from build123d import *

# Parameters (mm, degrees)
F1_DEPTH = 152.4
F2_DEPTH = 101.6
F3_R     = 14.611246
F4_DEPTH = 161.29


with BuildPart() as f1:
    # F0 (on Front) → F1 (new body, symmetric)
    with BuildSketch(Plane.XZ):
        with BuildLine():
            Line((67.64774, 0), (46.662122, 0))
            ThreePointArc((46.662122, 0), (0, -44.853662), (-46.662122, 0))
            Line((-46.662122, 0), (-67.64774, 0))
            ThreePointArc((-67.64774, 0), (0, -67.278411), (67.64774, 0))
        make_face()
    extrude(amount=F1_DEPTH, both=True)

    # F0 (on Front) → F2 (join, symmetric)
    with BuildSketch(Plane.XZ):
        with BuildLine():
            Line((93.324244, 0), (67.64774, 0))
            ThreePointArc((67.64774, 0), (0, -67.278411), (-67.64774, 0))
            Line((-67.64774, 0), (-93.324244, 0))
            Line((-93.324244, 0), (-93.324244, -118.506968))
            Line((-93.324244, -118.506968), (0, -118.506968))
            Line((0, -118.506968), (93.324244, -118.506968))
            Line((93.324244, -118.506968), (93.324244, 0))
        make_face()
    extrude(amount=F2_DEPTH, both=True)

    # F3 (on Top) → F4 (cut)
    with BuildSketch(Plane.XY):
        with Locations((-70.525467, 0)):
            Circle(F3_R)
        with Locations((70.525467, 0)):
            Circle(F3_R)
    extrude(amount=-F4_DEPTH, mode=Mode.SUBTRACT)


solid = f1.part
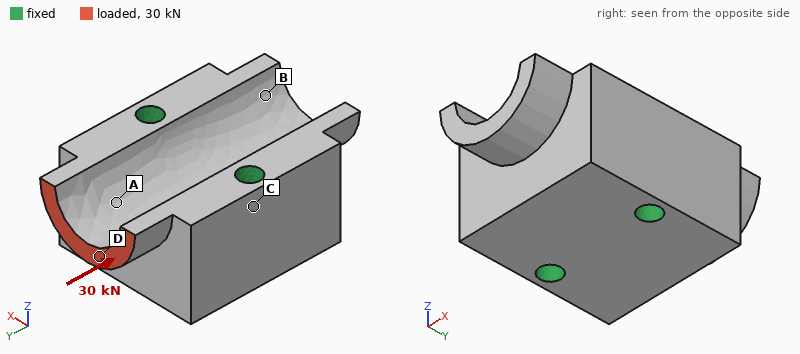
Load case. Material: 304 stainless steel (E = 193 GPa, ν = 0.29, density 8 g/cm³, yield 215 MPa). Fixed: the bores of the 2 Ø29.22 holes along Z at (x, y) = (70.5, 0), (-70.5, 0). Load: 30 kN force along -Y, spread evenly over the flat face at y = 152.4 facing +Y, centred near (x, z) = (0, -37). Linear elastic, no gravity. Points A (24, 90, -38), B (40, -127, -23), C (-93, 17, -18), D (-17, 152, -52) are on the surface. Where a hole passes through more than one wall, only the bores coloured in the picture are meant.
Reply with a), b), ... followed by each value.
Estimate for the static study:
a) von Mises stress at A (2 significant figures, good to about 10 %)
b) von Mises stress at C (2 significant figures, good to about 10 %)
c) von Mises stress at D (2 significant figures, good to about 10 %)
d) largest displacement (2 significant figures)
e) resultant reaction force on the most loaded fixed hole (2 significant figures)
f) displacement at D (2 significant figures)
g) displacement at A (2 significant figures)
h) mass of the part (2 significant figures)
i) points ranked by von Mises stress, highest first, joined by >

a) 5.2 MPa
b) 2.6 MPa
c) 7.4 MPa
d) 6.1 µm
e) 15 kN
f) 4.2 µm
g) 2.3 µm
h) 33 kg
i) D > A > C > B
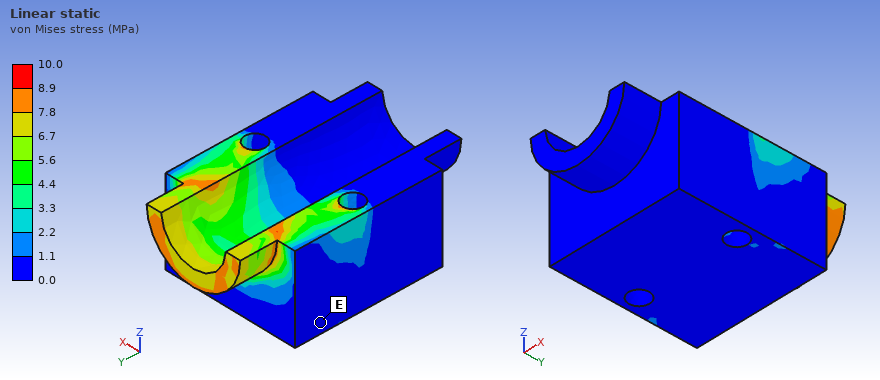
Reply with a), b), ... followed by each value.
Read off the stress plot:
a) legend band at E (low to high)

a) 0.0 to 1.1 MPa
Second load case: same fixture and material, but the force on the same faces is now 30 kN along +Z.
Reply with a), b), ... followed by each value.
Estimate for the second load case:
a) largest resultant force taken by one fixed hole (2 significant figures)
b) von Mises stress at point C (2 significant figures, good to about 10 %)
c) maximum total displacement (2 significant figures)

a) 15 kN
b) 8.3 MPa
c) 49 µm
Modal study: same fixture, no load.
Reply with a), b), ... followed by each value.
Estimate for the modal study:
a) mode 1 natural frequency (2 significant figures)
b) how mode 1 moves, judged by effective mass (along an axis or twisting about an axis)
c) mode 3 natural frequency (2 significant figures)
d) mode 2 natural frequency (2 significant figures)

a) 3900 Hz
b) twisting about X
c) 4300 Hz
d) 4200 Hz
